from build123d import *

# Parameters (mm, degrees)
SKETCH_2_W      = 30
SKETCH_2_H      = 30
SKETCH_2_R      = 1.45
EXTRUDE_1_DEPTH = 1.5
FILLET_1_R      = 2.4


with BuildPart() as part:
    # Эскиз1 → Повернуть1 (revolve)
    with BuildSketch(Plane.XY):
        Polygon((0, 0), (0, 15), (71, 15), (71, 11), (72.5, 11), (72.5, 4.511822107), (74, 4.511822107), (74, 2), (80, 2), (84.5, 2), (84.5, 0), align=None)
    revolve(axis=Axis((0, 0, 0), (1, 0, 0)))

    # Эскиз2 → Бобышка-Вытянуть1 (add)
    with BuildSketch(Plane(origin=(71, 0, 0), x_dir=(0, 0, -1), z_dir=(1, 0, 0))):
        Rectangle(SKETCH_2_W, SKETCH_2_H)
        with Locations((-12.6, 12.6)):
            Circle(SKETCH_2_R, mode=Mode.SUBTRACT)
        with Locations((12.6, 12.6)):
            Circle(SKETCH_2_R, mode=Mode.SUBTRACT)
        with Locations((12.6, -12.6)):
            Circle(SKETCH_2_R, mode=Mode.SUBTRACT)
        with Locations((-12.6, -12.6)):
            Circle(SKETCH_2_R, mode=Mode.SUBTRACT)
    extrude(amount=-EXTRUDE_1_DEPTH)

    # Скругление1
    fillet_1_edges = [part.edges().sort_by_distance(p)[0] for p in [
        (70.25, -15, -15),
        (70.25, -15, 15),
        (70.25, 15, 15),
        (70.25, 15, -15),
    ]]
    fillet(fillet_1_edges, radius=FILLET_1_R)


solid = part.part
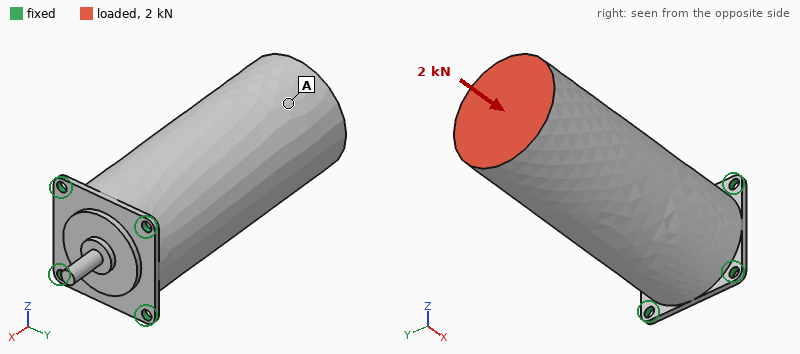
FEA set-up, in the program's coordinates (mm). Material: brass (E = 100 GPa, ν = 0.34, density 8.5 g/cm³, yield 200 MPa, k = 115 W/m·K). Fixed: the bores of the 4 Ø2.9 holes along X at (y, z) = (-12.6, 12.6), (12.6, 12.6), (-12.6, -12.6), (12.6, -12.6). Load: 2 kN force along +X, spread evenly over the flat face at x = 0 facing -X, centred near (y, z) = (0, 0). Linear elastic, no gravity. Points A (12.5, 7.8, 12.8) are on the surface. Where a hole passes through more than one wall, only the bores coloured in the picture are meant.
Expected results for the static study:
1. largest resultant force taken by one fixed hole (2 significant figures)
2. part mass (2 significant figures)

550 N
440 g
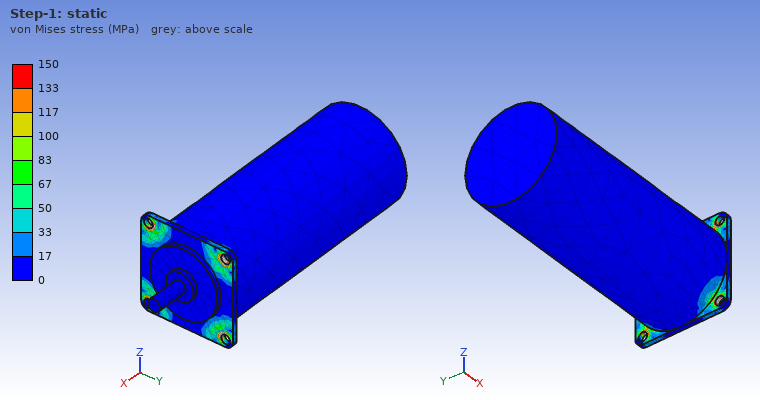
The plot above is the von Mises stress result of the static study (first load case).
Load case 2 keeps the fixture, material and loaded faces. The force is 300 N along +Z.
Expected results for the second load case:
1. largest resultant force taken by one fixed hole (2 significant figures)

500 N
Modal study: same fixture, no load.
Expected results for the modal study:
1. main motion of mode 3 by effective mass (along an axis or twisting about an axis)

along X
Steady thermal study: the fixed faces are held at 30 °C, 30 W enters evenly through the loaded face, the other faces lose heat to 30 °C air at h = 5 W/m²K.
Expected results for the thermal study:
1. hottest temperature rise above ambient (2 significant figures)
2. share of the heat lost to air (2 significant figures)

44 K
3.8 %
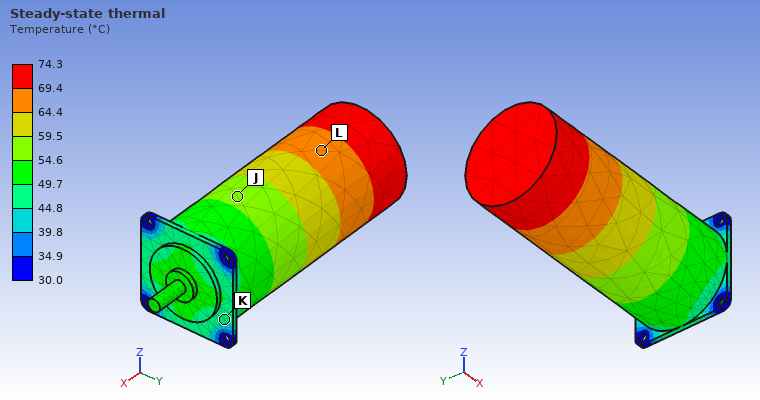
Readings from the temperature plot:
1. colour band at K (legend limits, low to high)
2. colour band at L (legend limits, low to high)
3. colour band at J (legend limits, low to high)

44.8 to 49.7 °C
64.4 to 69.4 °C
54.6 to 59.5 °C
